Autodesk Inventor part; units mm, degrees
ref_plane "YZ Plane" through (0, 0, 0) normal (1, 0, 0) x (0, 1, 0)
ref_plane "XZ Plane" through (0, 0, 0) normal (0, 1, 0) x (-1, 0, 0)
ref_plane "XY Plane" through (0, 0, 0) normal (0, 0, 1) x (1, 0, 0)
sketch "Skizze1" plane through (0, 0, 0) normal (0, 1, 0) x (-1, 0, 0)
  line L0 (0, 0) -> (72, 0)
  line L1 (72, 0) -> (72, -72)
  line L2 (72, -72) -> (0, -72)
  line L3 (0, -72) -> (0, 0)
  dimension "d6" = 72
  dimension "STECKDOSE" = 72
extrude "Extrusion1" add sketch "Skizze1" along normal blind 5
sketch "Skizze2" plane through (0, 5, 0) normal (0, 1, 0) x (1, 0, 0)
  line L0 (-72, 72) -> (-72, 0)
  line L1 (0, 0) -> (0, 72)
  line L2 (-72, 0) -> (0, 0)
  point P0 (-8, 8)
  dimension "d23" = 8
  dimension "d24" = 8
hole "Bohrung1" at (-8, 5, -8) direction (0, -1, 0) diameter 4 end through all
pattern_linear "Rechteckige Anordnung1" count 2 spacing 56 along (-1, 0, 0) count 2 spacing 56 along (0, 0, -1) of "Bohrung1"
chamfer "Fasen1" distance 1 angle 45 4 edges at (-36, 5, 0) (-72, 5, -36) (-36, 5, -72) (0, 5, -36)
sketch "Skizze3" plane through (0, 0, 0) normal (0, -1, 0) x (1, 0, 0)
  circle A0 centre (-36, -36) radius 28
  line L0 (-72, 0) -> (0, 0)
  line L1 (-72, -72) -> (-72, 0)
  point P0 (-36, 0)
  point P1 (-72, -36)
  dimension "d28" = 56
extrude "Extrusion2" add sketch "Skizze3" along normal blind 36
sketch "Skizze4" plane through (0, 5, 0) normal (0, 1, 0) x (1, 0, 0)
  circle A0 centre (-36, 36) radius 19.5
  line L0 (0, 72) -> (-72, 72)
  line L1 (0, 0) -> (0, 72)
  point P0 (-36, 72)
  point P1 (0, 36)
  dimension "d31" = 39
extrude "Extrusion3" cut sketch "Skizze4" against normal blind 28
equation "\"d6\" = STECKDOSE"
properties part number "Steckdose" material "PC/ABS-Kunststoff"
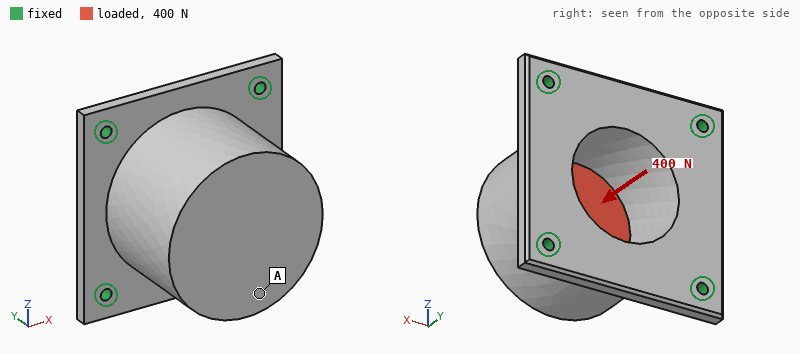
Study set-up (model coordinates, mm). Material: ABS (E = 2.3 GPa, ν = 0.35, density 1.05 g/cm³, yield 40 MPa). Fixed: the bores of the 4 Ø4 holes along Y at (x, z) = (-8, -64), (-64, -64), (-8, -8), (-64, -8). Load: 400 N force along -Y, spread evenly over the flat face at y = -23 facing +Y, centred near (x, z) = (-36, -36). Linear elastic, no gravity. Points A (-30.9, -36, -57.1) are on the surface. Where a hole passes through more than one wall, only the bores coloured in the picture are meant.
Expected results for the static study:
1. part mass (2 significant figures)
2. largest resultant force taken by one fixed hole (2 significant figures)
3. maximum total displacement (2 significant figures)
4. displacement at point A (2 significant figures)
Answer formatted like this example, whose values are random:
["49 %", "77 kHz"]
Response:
["85 g", "110 N", "83 µm", "74 µm"]
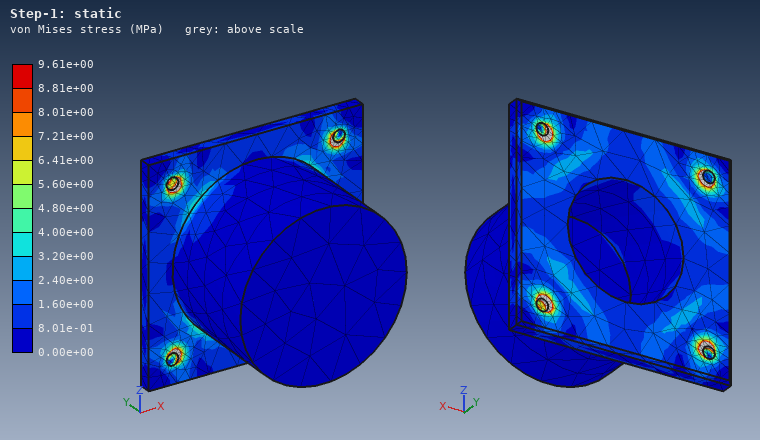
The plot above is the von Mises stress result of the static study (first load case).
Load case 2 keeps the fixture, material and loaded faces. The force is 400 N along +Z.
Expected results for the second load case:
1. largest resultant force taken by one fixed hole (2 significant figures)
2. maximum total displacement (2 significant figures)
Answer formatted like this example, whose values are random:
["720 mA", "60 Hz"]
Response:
["150 N", "0.16 mm"]
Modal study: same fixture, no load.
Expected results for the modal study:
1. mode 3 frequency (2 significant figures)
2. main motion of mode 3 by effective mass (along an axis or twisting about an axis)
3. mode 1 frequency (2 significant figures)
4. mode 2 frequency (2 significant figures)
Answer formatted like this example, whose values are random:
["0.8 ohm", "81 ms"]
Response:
["1300 Hz", "along Y", "1100 Hz", "1100 Hz"]
